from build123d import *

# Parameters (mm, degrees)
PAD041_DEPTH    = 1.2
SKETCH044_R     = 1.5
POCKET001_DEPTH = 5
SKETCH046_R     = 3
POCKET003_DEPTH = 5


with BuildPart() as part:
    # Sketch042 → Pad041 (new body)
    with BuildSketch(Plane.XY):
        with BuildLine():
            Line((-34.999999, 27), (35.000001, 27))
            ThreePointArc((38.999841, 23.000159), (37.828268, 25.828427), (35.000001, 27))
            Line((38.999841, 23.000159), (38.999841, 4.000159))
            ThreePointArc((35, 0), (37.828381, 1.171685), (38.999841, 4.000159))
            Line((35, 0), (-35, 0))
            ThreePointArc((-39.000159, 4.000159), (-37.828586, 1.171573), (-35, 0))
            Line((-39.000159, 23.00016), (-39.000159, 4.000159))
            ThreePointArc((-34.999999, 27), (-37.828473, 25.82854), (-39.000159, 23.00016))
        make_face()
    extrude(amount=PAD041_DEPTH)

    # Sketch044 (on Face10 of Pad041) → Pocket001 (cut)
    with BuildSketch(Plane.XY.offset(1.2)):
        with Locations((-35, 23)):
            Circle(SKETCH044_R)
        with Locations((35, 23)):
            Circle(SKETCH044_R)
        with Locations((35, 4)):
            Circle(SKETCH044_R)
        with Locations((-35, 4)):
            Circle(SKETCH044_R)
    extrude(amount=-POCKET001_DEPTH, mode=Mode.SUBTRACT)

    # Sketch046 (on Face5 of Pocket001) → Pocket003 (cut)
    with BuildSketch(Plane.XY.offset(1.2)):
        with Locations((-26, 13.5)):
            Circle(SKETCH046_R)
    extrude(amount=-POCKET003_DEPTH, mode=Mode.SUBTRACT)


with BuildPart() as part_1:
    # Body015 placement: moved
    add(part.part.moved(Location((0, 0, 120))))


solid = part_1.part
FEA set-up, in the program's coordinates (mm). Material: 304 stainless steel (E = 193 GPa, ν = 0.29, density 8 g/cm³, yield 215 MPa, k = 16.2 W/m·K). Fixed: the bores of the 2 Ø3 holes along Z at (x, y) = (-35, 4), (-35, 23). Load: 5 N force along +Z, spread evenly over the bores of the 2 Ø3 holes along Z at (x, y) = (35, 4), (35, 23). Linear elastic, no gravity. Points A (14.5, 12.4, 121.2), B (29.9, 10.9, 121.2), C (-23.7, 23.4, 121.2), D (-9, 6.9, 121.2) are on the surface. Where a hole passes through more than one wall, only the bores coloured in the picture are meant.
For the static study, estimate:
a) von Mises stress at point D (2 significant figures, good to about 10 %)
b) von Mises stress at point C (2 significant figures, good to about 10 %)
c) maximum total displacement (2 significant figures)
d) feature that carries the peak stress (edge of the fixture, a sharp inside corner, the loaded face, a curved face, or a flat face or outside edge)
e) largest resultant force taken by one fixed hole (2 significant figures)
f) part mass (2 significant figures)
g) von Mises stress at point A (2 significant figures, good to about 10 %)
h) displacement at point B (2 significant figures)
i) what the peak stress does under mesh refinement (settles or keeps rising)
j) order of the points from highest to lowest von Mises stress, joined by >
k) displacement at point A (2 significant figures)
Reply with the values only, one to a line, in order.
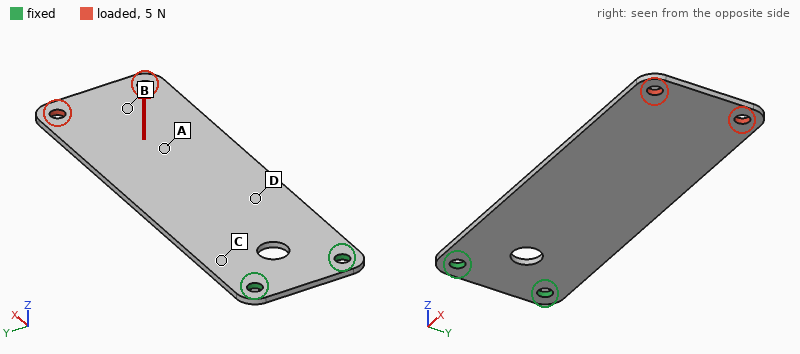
33 MPa
52 MPa
0.86 mm
edge of the fixture
2.5 N
20 g
16 MPa
0.71 mm
keeps rising
C > D > A > B
0.46 mm
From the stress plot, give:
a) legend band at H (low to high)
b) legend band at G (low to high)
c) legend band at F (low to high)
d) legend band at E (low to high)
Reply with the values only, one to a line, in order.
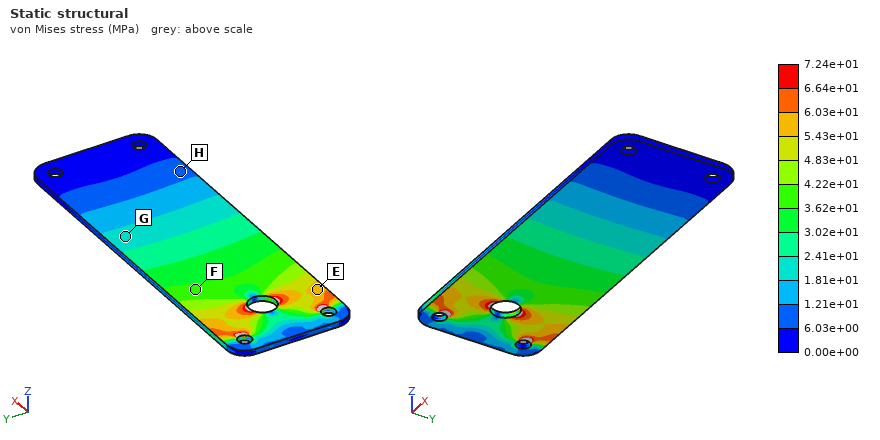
6.03e+00 to 1.21e+01 MPa
1.81e+01 to 2.41e+01 MPa
3.62e+01 to 4.22e+01 MPa
5.43e+01 to 6.03e+01 MPa
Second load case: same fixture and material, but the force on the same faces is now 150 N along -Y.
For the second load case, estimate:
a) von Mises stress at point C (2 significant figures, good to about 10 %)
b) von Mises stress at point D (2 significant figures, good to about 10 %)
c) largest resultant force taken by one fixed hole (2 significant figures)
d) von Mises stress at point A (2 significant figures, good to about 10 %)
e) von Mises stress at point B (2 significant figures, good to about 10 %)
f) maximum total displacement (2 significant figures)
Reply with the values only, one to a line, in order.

44 MPa
24 MPa
520 N
12 MPa
11 MPa
57 µm
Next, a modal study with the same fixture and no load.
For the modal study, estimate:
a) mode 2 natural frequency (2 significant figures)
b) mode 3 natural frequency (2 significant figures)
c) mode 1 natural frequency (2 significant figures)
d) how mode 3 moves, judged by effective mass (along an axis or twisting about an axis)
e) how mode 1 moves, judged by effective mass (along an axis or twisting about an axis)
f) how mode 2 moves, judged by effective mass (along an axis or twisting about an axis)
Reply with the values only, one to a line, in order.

1000 Hz
1100 Hz
170 Hz
along Z
along Z
twisting about X
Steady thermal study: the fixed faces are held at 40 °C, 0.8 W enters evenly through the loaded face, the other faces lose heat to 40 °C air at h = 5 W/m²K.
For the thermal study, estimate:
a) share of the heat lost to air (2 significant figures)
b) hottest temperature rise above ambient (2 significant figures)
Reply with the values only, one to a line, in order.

67 %
62 K
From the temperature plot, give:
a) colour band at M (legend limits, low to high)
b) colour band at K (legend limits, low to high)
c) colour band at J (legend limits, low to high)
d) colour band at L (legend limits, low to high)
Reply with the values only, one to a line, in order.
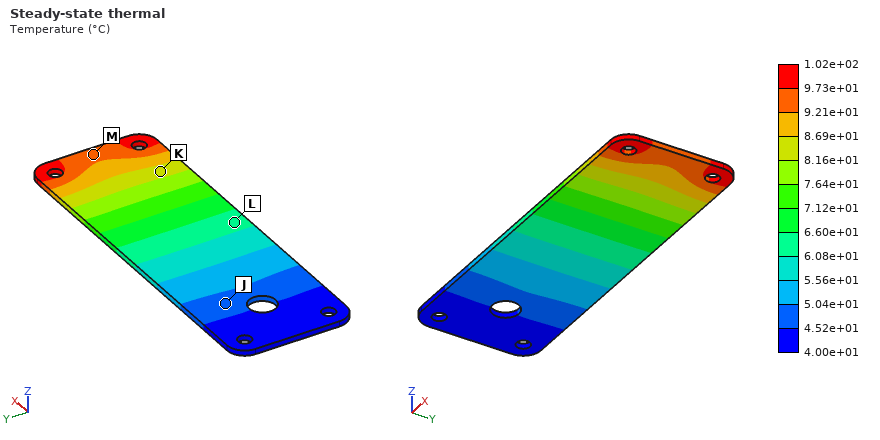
9.21e+01 to 9.73e+01 °C
8.16e+01 to 8.69e+01 °C
4.52e+01 to 5.04e+01 °C
6.08e+01 to 6.60e+01 °C
